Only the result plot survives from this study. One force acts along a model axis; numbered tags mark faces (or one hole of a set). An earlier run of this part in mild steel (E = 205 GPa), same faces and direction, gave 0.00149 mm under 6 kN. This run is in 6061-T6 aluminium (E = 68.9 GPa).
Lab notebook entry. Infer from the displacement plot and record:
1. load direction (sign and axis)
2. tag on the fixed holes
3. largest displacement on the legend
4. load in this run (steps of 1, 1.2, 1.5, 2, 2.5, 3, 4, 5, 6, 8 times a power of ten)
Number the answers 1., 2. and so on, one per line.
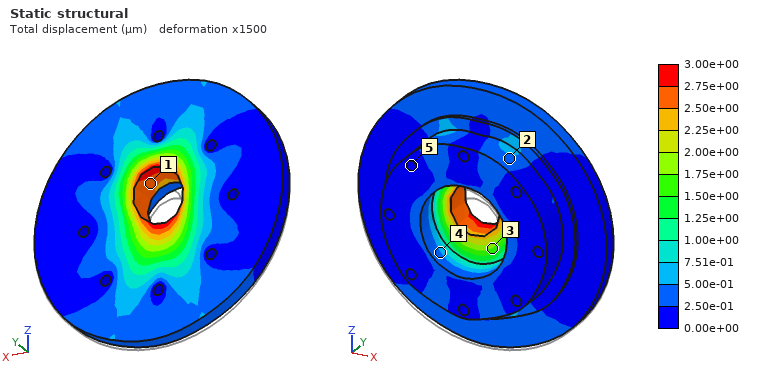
1. +Z
2. 5
3. 3.00e+00 µm
4. 4 kN
